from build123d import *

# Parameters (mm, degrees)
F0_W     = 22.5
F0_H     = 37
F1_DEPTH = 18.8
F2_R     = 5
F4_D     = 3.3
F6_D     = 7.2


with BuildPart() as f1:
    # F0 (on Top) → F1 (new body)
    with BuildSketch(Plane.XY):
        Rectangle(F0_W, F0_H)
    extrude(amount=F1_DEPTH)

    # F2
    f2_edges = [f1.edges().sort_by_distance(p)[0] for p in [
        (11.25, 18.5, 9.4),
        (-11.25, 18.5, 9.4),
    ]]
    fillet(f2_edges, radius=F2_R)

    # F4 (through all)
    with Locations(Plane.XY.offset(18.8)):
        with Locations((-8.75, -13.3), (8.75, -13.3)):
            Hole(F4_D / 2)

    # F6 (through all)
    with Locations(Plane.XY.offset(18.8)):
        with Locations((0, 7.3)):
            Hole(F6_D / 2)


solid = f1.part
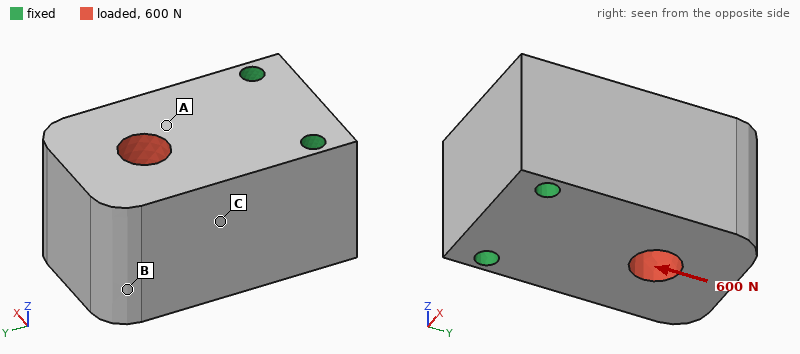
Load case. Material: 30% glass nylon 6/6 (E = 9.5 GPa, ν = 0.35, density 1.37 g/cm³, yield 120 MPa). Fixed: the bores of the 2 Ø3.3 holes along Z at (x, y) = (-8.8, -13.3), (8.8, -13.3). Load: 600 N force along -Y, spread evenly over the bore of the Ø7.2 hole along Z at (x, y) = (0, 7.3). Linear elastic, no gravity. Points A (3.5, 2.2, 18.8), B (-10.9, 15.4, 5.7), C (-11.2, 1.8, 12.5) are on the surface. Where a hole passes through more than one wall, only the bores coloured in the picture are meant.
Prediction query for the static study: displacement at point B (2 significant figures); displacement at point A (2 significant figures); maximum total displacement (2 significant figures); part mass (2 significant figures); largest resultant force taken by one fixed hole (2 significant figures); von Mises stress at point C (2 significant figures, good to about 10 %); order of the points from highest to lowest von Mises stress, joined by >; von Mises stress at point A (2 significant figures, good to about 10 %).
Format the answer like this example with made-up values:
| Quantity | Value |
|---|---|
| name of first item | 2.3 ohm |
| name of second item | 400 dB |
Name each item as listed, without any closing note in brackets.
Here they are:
| Quantity | Value |
|---|---|
| displacement at point B | 3.1 µm |
| displacement at point A | 2.8 µm |
| maximum total displacement | 5.3 µm |
| part mass | 20 g |
| largest resultant force taken by one fixed hole | 310 N |
| von Mises stress at point C | 1.0 MPa |
| order of the points from highest to lowest von Mises stress, joined by > | A > C > B |
| von Mises stress at point A | 1.9 MPa |
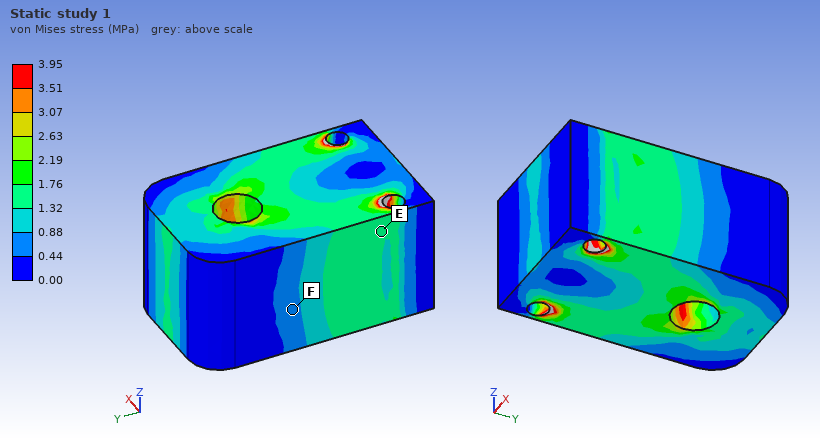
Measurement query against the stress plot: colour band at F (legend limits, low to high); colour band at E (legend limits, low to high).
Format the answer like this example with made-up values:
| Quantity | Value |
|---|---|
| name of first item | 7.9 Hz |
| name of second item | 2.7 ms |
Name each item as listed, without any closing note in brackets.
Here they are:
| Quantity | Value |
|---|---|
| colour band at F | 0.44 to 0.88 MPa |
| colour band at E | 1.32 to 1.76 MPa |
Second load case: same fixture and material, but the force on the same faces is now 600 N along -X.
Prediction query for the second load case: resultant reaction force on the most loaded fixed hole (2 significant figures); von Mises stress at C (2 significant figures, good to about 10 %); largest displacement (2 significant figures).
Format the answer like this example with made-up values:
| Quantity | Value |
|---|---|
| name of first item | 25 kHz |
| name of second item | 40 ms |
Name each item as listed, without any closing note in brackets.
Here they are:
| Quantity | Value |
|---|---|
| resultant reaction force on the most loaded fixed hole | 730 N |
| von Mises stress at C | 2.6 MPa |
| largest displacement | 29 µm |
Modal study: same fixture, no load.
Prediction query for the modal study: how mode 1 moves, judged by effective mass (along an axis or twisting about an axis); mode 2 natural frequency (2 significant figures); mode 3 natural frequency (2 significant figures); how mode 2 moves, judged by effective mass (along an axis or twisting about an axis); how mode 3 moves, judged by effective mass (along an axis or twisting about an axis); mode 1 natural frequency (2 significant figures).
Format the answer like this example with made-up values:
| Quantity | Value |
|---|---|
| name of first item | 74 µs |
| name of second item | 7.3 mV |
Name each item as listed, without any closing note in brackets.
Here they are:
| Quantity | Value |
|---|---|
| how mode 1 moves, judged by effective mass | along Z |
| mode 2 natural frequency | 7600 Hz |
| mode 3 natural frequency | 12 kHz |
| how mode 2 moves, judged by effective mass | along X |
| how mode 3 moves, judged by effective mass | twisting about Y |
| mode 1 natural frequency | 6200 Hz |
